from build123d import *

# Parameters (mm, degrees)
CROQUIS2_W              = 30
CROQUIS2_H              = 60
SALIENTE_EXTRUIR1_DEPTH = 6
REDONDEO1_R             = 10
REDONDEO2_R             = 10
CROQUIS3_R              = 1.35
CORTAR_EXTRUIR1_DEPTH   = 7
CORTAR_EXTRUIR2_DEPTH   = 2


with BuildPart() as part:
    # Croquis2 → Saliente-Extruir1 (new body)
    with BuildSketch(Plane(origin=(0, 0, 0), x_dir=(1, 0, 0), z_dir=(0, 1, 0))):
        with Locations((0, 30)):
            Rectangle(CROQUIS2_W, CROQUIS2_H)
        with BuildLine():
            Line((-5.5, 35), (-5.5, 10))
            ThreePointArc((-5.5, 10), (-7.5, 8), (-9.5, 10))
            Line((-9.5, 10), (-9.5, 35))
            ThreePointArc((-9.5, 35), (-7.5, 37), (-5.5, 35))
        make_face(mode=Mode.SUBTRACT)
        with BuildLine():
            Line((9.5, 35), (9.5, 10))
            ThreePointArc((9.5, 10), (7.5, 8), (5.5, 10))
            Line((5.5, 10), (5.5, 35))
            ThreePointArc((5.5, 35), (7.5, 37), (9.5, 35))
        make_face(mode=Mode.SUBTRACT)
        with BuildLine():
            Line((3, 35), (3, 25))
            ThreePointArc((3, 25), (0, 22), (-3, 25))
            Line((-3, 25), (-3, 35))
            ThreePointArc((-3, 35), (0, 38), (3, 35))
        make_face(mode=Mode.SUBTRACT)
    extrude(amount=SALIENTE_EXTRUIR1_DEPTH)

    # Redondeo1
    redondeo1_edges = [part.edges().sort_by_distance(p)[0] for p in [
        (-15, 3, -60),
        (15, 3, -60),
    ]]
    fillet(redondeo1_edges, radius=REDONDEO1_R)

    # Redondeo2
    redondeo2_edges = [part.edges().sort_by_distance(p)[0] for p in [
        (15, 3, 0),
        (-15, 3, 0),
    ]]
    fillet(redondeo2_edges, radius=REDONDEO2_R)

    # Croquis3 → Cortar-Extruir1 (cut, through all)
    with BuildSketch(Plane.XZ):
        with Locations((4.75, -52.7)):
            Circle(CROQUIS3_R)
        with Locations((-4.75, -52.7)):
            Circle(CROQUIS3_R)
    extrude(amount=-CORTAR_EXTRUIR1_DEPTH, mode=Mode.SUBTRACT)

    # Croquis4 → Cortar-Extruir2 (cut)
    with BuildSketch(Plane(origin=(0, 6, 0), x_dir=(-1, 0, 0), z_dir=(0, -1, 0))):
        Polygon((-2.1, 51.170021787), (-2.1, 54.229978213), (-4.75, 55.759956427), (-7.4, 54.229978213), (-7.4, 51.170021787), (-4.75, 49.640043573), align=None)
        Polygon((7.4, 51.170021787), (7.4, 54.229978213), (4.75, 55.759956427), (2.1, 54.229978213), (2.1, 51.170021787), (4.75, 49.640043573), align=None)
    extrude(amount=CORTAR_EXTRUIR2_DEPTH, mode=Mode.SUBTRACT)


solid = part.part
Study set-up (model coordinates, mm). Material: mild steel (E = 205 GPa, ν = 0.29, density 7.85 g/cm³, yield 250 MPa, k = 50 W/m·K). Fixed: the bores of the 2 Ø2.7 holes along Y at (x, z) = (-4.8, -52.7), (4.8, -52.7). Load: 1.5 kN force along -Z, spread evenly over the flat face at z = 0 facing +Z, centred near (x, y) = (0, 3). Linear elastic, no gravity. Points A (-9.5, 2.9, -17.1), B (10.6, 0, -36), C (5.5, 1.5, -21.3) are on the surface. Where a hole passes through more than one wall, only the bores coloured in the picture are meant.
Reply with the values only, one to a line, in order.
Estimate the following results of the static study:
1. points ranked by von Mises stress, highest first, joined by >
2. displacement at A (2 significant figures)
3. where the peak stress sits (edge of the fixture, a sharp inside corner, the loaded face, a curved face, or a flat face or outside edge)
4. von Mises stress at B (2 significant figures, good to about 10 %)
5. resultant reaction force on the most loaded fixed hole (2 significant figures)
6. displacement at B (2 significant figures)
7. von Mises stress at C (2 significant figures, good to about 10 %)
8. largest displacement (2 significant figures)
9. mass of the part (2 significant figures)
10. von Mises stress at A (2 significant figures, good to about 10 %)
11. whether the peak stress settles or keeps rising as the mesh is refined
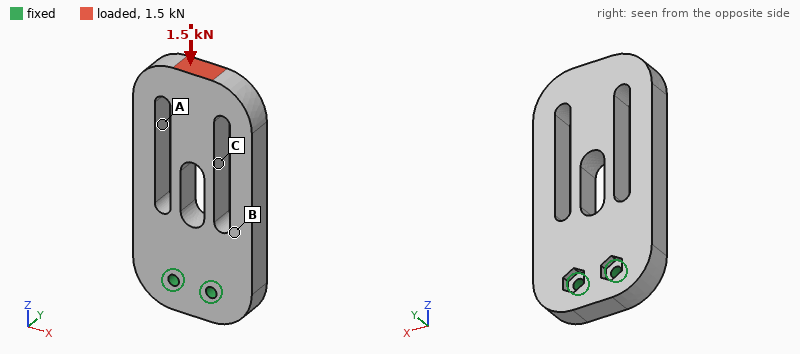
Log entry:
C > A > B
5.2 µm
edge of the fixture
8.5 MPa
750 N
2.2 µm
28 MPa
8.7 µm
65 g
19 MPa
keeps rising
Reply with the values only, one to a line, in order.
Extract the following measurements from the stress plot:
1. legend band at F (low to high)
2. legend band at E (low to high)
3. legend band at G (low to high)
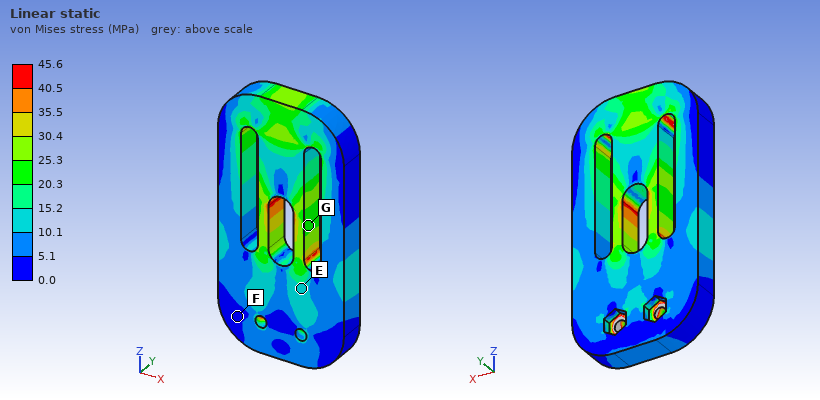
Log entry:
0.0 to 5.1 MPa
10.1 to 15.2 MPa
20.3 to 25.3 MPa
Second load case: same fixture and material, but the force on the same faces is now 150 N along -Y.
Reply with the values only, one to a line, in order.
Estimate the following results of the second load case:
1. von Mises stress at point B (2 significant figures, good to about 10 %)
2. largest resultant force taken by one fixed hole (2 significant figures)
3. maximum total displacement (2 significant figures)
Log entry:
50 MPa
86 N
0.11 mm
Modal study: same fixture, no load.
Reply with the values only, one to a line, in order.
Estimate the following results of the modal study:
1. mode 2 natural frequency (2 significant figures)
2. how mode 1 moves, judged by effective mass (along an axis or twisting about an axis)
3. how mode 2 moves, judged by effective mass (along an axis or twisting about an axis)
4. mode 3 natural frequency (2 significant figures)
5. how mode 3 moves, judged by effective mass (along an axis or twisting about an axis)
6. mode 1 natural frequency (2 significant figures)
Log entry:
3600 Hz
along Y
along X
4800 Hz
twisting about Z
1500 Hz
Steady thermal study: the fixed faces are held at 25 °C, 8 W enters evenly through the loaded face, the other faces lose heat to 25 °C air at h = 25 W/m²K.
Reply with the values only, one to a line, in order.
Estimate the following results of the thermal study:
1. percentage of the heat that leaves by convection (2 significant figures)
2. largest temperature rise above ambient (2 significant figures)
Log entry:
34 %
62 K
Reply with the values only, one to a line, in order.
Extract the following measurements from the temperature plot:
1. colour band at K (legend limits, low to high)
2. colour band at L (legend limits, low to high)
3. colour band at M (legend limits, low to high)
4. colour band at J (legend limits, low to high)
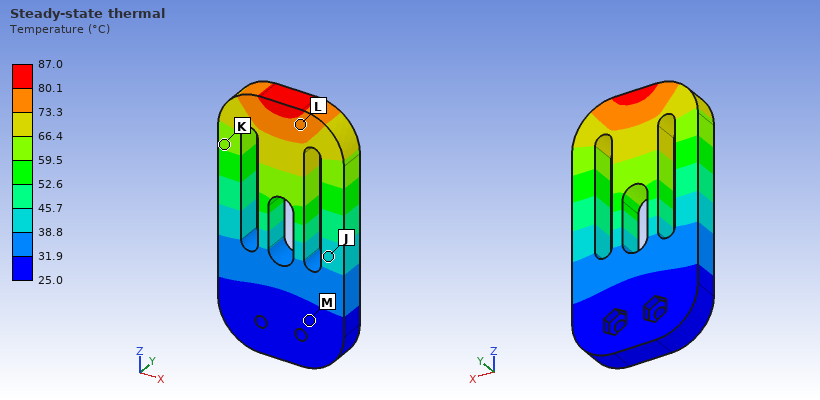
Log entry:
59.5 to 66.4 °C
73.3 to 80.1 °C
25.0 to 31.9 °C
38.8 to 45.7 °C
